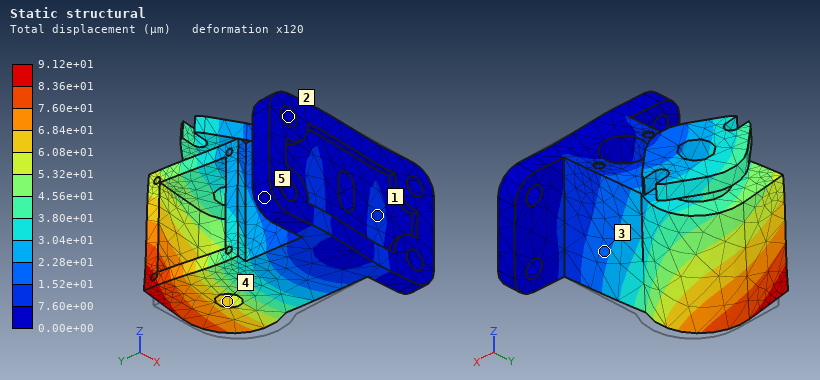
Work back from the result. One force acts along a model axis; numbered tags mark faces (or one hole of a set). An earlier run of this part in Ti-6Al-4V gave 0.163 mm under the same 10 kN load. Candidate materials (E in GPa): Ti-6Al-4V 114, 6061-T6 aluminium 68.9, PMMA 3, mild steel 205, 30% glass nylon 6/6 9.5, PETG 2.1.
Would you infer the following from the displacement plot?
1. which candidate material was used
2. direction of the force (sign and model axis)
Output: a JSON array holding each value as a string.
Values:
["mild steel", "-X"]
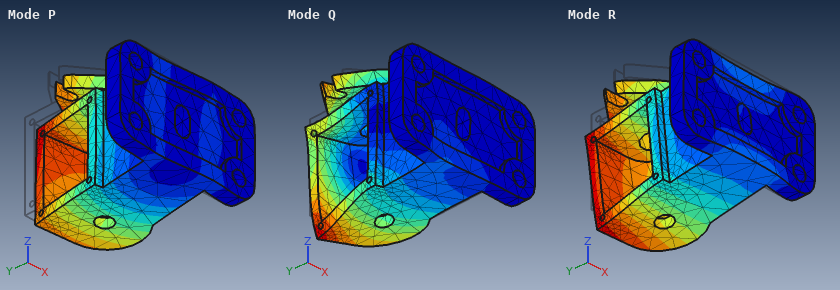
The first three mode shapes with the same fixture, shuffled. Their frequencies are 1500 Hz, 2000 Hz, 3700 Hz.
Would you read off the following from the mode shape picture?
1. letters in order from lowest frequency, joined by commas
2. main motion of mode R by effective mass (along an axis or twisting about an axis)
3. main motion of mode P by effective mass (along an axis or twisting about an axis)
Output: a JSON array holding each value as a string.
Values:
["R, P, Q", "along Z", "along X"]
